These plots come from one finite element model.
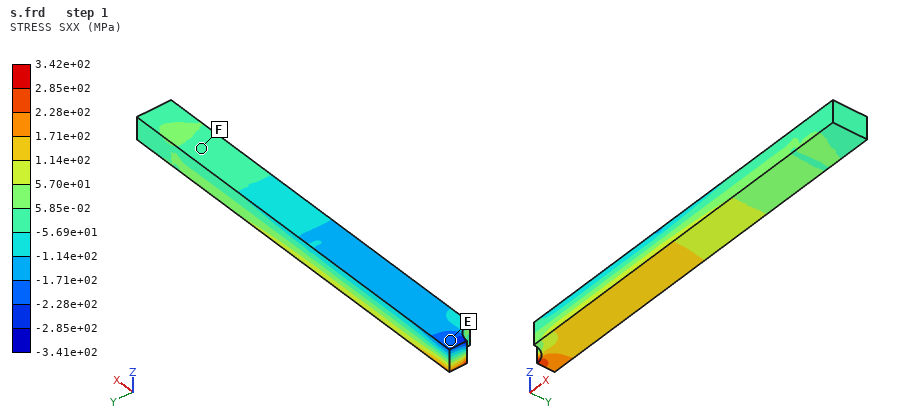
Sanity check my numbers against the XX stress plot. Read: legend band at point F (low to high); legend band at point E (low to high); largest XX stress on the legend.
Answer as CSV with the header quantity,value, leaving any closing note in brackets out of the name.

quantity,value
legend band at point F,-5.69e+01 to 5.85e-02 MPa
legend band at point E,-2.28e+02 to -1.71e+02 MPa
largest XX stress on the legend,3.42e+02 MPa
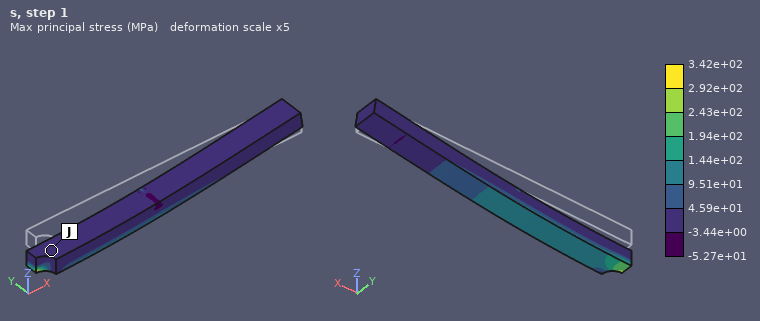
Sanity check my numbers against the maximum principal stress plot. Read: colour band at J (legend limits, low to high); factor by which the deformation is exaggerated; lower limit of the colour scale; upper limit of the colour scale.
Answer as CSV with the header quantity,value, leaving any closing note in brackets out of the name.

quantity,value
colour band at J,-3.44e+00 to 4.59e+01 MPa
factor by which the deformation is exaggerated,5
lower limit of the colour scale,-5.27e+01 MPa
upper limit of the colour scale,3.42e+02 MPa
